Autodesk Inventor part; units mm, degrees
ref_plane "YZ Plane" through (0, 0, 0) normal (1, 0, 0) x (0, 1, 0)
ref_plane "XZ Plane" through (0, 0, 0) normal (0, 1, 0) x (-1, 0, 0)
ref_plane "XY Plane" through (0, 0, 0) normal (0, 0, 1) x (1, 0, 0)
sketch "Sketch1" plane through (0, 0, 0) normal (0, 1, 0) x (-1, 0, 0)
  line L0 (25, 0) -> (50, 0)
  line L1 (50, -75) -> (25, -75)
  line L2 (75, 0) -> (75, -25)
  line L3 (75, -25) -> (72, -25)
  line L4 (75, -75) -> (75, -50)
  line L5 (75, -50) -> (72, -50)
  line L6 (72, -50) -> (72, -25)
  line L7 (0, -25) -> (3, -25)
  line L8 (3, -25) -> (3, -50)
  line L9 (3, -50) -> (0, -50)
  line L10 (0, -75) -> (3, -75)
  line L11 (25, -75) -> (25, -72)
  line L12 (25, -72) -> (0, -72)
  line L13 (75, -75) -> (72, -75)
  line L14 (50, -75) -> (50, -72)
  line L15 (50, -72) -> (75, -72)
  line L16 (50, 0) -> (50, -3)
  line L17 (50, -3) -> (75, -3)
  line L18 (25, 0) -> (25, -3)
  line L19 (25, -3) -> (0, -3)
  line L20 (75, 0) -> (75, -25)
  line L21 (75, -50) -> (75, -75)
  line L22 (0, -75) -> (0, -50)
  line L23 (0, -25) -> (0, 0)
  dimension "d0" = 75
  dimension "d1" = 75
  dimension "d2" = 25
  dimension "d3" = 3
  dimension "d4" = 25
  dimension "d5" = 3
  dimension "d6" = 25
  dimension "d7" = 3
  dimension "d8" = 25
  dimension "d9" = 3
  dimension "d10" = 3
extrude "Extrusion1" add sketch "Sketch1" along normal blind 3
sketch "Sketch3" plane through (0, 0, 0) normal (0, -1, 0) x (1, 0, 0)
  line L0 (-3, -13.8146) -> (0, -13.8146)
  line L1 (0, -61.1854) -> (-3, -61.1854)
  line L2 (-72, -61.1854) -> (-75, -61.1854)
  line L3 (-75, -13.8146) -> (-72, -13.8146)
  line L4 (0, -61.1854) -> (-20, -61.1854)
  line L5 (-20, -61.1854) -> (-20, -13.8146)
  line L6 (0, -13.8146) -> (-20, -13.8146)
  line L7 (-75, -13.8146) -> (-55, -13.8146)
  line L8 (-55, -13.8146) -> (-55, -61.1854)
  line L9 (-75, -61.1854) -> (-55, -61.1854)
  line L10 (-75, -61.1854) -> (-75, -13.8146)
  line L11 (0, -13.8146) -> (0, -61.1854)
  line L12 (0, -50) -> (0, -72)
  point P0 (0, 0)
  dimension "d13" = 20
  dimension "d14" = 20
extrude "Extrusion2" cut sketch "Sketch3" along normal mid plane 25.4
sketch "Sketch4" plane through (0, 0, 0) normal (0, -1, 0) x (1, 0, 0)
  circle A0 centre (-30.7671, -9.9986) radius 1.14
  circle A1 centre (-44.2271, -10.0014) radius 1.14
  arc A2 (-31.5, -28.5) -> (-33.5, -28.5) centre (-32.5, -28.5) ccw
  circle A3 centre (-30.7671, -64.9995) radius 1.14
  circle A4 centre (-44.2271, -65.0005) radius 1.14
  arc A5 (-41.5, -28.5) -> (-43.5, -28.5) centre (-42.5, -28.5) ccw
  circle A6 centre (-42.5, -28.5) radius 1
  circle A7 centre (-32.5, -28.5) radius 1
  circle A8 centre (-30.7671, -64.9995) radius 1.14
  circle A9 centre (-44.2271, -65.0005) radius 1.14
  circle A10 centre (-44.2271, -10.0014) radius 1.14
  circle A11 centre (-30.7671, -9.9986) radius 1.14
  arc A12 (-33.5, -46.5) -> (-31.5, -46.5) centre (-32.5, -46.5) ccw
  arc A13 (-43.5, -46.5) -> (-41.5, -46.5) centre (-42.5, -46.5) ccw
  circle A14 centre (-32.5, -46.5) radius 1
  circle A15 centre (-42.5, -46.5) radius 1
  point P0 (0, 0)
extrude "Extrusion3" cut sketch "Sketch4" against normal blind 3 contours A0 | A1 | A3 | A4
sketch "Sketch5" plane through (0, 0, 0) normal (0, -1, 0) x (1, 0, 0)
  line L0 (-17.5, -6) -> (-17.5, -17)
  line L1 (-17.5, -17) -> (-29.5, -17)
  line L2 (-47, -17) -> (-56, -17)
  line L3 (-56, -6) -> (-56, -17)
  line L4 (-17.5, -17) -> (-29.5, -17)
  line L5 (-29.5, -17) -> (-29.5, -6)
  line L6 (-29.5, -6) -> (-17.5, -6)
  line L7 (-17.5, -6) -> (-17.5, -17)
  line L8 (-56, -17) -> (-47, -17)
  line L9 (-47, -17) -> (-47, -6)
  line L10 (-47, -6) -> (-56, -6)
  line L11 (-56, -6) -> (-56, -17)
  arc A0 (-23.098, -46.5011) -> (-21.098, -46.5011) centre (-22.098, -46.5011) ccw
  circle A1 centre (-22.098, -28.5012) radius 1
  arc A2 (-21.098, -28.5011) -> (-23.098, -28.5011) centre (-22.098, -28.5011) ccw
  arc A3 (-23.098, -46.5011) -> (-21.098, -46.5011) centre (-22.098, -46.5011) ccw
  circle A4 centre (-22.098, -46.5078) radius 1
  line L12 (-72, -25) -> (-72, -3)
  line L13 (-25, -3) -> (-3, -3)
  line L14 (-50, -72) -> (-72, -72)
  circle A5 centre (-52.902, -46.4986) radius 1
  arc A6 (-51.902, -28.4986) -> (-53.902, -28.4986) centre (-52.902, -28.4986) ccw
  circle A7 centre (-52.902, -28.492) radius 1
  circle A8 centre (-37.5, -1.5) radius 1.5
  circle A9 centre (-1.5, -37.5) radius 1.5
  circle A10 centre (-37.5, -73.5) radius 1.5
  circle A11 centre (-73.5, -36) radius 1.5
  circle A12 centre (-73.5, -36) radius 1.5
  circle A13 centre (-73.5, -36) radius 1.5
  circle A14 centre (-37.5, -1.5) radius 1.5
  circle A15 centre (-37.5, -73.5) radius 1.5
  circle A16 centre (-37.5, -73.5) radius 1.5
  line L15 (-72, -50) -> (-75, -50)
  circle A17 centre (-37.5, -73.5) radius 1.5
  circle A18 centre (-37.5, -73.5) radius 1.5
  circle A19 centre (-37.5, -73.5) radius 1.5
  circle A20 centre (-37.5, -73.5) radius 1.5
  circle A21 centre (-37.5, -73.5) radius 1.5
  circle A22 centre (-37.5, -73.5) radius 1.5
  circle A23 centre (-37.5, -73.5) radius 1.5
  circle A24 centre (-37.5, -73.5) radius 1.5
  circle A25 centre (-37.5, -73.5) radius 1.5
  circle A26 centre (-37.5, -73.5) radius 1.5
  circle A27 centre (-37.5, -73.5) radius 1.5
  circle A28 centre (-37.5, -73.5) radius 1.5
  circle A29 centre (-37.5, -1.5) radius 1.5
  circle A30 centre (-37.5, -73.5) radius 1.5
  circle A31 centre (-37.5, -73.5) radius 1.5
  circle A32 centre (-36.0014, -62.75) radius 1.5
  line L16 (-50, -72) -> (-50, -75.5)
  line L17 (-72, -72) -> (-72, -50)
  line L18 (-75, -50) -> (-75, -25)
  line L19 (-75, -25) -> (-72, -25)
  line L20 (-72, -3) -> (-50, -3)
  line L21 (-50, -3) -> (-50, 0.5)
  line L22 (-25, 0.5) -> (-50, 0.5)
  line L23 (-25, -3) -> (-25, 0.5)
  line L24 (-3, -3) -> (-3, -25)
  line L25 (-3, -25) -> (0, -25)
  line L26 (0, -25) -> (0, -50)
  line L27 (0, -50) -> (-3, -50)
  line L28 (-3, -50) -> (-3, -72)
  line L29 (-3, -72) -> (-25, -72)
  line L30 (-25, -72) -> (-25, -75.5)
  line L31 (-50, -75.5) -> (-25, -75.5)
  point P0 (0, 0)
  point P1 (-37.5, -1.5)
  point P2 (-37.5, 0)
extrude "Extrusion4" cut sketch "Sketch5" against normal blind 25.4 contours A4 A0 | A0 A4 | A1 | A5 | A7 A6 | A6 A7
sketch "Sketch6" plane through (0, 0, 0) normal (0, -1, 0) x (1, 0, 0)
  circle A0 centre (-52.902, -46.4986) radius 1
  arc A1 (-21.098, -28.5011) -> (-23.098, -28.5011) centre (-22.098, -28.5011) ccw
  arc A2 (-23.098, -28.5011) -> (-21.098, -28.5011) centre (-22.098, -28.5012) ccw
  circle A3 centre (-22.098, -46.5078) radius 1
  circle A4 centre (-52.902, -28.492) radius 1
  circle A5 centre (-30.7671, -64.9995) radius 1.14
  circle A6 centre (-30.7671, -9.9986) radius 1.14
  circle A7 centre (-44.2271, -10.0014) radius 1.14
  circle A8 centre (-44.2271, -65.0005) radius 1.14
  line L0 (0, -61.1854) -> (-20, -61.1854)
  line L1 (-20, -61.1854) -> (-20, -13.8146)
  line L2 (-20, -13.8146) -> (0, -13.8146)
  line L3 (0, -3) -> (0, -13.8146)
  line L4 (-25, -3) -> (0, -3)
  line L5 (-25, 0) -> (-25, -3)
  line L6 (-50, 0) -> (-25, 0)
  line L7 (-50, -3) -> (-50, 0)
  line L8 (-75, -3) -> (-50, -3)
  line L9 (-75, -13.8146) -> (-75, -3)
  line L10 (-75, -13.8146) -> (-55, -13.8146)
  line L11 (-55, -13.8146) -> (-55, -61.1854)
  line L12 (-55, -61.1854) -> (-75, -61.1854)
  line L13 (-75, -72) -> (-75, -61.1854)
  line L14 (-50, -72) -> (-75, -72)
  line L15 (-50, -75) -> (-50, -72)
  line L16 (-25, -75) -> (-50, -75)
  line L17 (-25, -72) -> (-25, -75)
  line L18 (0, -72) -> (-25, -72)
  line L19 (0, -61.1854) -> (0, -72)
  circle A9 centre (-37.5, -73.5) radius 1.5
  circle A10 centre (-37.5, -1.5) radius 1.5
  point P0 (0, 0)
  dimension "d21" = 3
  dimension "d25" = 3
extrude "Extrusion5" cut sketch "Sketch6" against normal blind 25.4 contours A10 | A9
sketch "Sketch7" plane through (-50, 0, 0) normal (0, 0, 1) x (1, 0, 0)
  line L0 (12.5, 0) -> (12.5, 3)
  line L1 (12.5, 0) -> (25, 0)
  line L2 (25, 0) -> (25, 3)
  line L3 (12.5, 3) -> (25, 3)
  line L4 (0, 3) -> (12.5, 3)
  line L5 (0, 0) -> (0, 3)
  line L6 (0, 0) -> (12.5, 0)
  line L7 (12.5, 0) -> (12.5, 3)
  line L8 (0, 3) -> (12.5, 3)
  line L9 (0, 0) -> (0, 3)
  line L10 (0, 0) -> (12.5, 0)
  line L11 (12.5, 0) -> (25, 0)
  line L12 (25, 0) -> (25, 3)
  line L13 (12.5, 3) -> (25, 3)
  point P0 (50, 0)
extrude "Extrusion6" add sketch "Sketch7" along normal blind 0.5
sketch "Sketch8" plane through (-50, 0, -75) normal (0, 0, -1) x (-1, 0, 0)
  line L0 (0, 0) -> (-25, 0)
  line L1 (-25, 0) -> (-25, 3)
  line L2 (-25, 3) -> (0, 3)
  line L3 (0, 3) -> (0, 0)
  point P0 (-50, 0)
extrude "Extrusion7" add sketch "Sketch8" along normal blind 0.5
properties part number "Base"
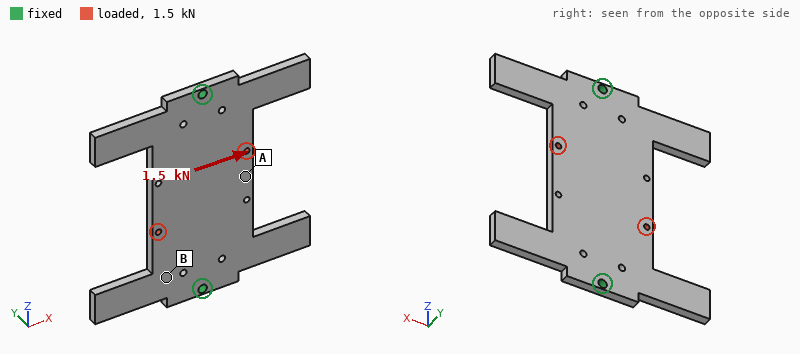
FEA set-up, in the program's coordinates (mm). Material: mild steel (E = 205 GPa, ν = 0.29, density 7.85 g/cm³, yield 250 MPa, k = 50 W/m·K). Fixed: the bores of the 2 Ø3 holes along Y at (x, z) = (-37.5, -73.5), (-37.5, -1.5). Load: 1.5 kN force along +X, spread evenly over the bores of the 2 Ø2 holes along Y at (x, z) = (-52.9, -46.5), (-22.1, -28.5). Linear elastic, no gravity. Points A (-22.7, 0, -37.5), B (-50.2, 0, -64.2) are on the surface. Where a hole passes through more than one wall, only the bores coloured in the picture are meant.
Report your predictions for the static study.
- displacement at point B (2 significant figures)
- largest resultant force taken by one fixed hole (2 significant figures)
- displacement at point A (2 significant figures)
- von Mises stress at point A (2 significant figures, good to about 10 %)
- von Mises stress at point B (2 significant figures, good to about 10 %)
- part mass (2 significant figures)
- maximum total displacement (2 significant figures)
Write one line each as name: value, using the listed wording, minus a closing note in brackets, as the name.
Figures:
displacement at point B: 3.8 µm
largest resultant force taken by one fixed hole: 750 N
displacement at point A: 7.6 µm
von Mises stress at point A: 26 MPa
von Mises stress at point B: 12 MPa
part mass: 80 g
maximum total displacement: 9.7 µm
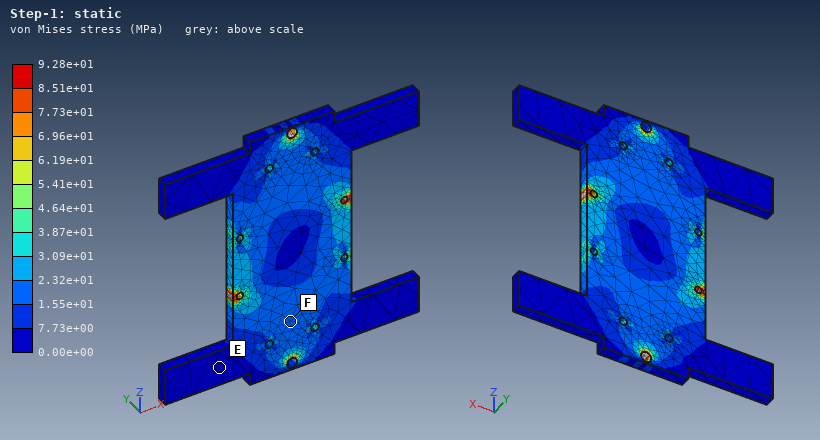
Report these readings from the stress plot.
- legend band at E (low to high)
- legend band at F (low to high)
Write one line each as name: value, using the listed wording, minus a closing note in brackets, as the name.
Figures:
legend band at E: 0.00e+00 to 7.73e+00 MPa
legend band at F: 1.55e+01 to 2.32e+01 MPa
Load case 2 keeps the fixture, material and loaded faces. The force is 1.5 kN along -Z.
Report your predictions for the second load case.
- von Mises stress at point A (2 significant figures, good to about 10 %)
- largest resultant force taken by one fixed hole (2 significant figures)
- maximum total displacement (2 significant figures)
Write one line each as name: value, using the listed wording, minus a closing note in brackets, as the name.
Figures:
von Mises stress at point A: 18 MPa
largest resultant force taken by one fixed hole: 750 N
maximum total displacement: 4.0 µm
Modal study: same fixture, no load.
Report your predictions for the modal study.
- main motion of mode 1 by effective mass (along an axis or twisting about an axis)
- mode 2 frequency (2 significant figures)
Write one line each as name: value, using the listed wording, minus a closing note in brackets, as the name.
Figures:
main motion of mode 1 by effective mass: twisting about Z
mode 2 frequency: 2100 Hz
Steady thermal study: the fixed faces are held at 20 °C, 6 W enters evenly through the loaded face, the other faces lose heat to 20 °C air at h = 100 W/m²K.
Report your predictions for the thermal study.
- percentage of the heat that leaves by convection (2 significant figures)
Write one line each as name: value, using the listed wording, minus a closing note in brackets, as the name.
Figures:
percentage of the heat that leaves by convection: 69 %
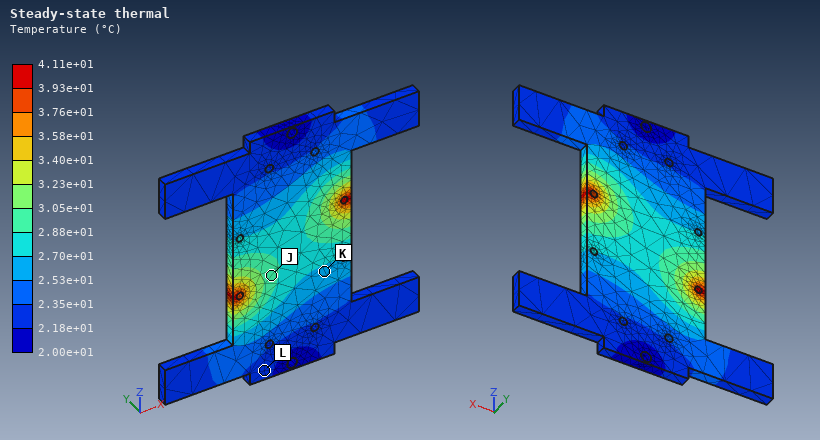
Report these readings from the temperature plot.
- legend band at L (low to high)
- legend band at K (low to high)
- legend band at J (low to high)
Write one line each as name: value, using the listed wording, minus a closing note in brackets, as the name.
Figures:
legend band at L: 2.18e+01 to 2.35e+01 °C
legend band at K: 2.53e+01 to 2.70e+01 °C
legend band at J: 2.88e+01 to 3.05e+01 °C
